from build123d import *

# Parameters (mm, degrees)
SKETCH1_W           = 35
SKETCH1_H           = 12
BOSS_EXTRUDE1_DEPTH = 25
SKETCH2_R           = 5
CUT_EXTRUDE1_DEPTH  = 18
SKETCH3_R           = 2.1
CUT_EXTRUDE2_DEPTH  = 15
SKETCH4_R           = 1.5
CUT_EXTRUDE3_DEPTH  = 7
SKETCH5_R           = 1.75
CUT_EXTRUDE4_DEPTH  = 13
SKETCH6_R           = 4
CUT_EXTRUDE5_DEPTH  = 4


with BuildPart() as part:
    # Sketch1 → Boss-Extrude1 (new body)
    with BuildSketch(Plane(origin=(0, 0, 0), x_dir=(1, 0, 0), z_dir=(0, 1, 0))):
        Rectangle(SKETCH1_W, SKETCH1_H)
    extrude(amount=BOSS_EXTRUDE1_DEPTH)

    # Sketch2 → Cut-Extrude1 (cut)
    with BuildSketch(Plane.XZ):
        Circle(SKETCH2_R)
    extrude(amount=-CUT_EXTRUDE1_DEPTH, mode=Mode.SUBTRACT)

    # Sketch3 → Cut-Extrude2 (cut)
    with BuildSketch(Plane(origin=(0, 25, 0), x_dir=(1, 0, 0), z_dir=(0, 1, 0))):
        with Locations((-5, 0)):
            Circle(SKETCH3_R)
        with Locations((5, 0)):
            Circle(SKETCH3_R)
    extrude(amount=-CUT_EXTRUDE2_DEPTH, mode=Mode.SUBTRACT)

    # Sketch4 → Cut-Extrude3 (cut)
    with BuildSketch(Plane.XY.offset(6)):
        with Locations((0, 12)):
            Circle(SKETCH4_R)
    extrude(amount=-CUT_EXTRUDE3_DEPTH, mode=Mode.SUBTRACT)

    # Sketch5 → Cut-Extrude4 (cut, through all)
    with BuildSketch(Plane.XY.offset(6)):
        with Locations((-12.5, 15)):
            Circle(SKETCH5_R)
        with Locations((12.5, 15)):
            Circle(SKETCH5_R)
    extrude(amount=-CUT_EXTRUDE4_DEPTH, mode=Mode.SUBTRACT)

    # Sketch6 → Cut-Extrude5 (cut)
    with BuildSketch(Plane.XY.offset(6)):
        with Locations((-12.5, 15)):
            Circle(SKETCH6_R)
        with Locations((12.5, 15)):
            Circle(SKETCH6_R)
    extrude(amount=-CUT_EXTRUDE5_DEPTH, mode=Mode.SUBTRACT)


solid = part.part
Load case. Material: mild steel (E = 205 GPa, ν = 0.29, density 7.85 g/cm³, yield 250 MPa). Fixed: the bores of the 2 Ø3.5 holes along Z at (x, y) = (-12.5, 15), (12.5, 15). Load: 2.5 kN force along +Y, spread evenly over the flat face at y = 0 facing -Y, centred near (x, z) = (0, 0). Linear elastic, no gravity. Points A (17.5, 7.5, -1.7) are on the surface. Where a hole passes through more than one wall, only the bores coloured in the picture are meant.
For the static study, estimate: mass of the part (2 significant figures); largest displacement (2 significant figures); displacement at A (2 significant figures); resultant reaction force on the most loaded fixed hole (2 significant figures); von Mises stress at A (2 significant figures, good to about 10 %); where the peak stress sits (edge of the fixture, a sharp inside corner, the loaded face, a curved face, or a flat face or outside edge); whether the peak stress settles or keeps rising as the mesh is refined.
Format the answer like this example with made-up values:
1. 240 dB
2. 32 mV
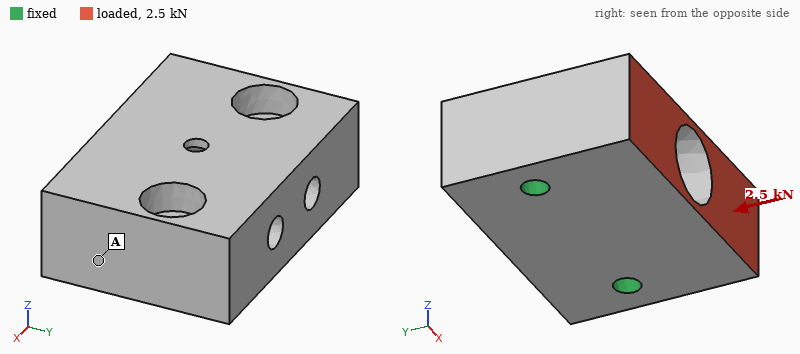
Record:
1. 64 g
2. 2.1 µm
3. 0.56 µm
4. 1.3 kN
5. 8.8 MPa
6. edge of the fixture
7. keeps rising
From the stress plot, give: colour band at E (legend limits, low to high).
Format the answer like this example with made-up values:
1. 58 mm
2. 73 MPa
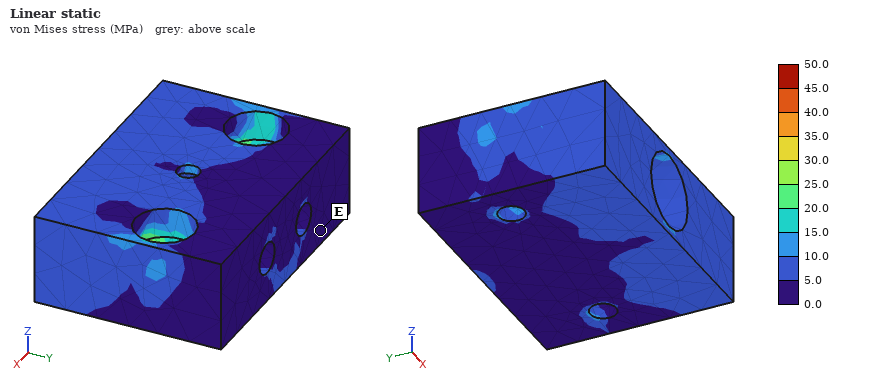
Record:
1. 0.0 to 5.0 MPa
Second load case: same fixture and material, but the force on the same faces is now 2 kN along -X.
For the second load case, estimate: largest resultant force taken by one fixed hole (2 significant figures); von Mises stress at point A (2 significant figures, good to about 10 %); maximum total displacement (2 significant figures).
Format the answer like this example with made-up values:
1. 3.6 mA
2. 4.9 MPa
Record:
1. 1.4 kN
2. 12 MPa
3. 4.0 µm
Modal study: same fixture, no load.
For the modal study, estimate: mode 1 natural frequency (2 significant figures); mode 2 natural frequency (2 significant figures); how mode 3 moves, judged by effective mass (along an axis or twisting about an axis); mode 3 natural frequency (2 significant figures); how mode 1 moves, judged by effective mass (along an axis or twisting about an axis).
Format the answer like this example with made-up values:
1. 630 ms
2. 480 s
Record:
1. 19 kHz
2. 26 kHz
3. along X
4. 32 kHz
5. along Z
